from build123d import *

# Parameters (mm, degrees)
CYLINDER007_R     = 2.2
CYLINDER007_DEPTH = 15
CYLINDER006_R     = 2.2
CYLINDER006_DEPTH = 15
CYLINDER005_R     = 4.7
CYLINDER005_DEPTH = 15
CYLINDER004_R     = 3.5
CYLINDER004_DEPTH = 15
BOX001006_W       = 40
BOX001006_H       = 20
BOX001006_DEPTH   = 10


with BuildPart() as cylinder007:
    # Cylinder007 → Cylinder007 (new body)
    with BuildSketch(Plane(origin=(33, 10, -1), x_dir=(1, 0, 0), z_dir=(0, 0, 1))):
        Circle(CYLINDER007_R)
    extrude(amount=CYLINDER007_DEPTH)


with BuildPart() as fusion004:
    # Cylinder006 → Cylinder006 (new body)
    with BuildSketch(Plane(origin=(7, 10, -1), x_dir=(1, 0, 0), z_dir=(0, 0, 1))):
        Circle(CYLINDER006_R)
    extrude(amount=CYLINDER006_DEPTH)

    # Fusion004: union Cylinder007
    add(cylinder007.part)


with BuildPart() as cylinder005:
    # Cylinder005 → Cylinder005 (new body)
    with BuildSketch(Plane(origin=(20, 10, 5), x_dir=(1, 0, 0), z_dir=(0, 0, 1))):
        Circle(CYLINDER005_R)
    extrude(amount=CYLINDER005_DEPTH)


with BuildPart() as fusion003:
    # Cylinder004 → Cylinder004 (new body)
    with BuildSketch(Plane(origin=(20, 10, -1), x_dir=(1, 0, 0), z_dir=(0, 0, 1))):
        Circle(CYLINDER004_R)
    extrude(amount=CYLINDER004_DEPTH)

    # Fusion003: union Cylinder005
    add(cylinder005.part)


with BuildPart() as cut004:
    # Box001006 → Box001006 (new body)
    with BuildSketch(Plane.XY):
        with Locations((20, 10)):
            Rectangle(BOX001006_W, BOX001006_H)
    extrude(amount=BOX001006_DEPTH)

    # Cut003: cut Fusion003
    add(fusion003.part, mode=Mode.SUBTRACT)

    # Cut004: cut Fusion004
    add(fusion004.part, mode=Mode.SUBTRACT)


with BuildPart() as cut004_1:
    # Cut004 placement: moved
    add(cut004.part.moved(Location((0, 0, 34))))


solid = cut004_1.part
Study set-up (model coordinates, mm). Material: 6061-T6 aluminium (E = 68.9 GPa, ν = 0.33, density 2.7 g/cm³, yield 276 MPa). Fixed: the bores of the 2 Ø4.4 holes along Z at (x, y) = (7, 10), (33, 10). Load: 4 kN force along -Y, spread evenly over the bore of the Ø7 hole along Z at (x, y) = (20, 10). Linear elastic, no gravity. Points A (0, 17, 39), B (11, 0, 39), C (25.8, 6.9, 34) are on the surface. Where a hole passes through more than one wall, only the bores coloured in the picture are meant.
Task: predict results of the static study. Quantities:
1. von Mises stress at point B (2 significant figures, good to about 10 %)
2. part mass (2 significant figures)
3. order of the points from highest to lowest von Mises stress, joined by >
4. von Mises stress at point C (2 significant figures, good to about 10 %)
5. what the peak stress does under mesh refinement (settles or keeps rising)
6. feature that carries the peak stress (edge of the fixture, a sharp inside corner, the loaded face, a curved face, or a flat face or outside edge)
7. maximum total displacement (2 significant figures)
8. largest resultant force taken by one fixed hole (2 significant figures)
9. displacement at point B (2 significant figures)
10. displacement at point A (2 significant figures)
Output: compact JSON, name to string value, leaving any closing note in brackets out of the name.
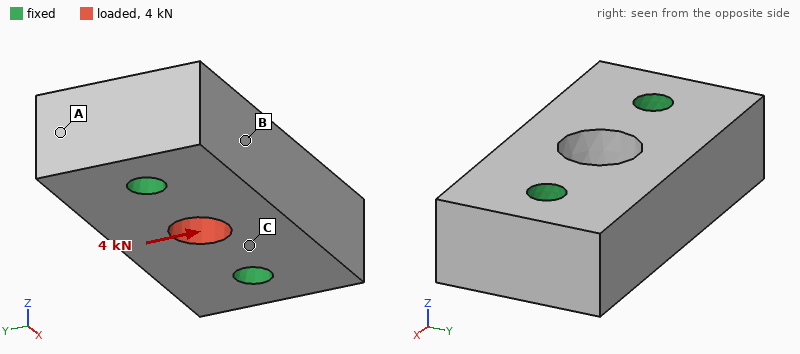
{"von Mises stress at point B": "13 MPa", "part mass": "19 g", "order of the points from highest to lowest von Mises stress, joined by >": "C > B > A", "von Mises stress at point C": "35 MPa", "what the peak stress does under mesh refinement": "keeps rising", "feature that carries the peak stress": "edge of the fixture", "maximum total displacement": "11 µm", "largest resultant force taken by one fixed hole": "2.0 kN", "displacement at point B": "4.3 µm", "displacement at point A": "2.1 µm"}
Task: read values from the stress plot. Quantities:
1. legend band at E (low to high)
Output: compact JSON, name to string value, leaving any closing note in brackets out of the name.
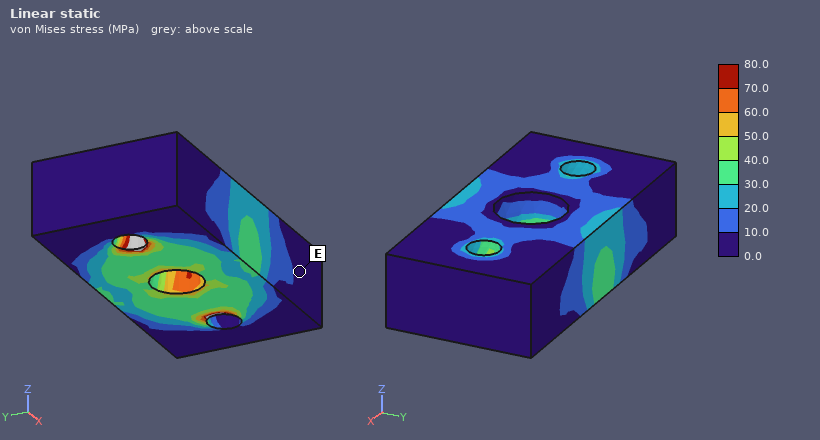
{"legend band at E": "0.0 to 10.0 MPa"}
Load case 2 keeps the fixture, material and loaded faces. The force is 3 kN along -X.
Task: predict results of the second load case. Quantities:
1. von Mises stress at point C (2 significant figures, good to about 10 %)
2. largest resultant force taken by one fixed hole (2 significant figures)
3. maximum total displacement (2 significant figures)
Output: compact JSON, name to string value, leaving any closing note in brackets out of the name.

{"von Mises stress at point C": "23 MPa", "largest resultant force taken by one fixed hole": "1.5 kN", "maximum total displacement": "3.5 µm"}
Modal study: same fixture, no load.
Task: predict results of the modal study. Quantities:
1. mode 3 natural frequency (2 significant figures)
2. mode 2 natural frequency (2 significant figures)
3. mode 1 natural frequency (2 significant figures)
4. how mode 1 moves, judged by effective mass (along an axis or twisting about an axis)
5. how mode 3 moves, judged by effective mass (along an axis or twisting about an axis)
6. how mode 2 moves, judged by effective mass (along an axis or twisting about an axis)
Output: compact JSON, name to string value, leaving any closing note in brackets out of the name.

{"mode 3 natural frequency": "49 kHz", "mode 2 natural frequency": "41 kHz", "mode 1 natural frequency": "39 kHz", "how mode 1 moves, judged by effective mass": "twisting about X", "how mode 3 moves, judged by effective mass": "along Y", "how mode 2 moves, judged by effective mass": "along Z"}
